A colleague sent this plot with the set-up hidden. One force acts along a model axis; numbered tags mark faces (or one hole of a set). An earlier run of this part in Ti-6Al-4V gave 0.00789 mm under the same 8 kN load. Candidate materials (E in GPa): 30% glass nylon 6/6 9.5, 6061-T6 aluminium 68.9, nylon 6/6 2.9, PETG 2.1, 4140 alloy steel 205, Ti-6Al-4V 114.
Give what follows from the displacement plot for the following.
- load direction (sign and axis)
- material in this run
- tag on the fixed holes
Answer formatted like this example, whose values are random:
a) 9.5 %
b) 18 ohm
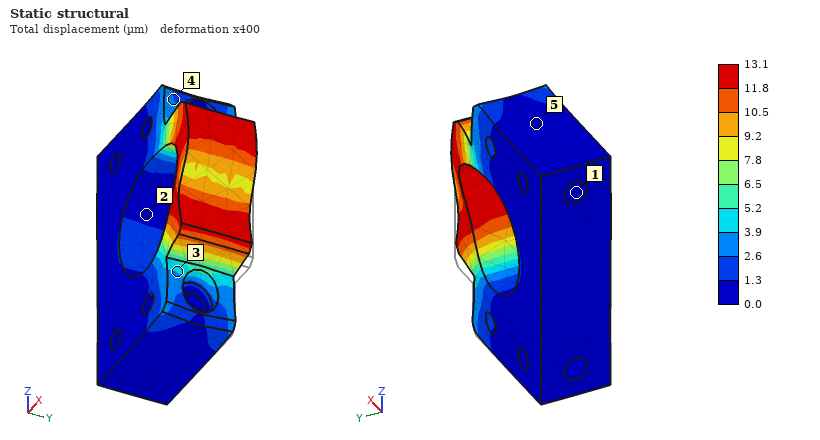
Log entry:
a) +Z
b) 6061-T6 aluminium
c) 1
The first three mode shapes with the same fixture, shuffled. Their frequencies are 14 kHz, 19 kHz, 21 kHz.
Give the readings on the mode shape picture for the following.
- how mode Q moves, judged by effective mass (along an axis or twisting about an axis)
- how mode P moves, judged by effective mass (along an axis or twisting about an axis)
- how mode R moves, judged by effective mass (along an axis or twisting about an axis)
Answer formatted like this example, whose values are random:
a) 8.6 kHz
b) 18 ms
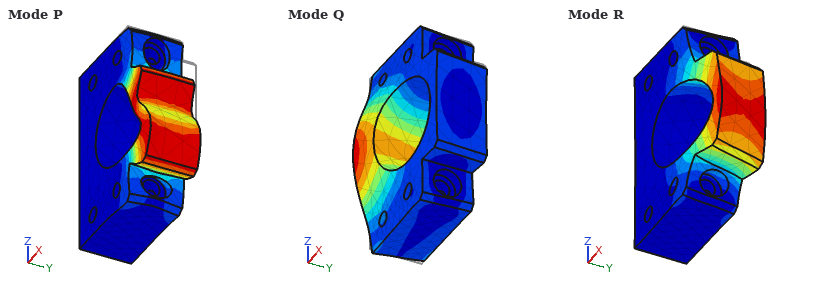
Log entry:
a) along Y
b) along Z
c) along Y
